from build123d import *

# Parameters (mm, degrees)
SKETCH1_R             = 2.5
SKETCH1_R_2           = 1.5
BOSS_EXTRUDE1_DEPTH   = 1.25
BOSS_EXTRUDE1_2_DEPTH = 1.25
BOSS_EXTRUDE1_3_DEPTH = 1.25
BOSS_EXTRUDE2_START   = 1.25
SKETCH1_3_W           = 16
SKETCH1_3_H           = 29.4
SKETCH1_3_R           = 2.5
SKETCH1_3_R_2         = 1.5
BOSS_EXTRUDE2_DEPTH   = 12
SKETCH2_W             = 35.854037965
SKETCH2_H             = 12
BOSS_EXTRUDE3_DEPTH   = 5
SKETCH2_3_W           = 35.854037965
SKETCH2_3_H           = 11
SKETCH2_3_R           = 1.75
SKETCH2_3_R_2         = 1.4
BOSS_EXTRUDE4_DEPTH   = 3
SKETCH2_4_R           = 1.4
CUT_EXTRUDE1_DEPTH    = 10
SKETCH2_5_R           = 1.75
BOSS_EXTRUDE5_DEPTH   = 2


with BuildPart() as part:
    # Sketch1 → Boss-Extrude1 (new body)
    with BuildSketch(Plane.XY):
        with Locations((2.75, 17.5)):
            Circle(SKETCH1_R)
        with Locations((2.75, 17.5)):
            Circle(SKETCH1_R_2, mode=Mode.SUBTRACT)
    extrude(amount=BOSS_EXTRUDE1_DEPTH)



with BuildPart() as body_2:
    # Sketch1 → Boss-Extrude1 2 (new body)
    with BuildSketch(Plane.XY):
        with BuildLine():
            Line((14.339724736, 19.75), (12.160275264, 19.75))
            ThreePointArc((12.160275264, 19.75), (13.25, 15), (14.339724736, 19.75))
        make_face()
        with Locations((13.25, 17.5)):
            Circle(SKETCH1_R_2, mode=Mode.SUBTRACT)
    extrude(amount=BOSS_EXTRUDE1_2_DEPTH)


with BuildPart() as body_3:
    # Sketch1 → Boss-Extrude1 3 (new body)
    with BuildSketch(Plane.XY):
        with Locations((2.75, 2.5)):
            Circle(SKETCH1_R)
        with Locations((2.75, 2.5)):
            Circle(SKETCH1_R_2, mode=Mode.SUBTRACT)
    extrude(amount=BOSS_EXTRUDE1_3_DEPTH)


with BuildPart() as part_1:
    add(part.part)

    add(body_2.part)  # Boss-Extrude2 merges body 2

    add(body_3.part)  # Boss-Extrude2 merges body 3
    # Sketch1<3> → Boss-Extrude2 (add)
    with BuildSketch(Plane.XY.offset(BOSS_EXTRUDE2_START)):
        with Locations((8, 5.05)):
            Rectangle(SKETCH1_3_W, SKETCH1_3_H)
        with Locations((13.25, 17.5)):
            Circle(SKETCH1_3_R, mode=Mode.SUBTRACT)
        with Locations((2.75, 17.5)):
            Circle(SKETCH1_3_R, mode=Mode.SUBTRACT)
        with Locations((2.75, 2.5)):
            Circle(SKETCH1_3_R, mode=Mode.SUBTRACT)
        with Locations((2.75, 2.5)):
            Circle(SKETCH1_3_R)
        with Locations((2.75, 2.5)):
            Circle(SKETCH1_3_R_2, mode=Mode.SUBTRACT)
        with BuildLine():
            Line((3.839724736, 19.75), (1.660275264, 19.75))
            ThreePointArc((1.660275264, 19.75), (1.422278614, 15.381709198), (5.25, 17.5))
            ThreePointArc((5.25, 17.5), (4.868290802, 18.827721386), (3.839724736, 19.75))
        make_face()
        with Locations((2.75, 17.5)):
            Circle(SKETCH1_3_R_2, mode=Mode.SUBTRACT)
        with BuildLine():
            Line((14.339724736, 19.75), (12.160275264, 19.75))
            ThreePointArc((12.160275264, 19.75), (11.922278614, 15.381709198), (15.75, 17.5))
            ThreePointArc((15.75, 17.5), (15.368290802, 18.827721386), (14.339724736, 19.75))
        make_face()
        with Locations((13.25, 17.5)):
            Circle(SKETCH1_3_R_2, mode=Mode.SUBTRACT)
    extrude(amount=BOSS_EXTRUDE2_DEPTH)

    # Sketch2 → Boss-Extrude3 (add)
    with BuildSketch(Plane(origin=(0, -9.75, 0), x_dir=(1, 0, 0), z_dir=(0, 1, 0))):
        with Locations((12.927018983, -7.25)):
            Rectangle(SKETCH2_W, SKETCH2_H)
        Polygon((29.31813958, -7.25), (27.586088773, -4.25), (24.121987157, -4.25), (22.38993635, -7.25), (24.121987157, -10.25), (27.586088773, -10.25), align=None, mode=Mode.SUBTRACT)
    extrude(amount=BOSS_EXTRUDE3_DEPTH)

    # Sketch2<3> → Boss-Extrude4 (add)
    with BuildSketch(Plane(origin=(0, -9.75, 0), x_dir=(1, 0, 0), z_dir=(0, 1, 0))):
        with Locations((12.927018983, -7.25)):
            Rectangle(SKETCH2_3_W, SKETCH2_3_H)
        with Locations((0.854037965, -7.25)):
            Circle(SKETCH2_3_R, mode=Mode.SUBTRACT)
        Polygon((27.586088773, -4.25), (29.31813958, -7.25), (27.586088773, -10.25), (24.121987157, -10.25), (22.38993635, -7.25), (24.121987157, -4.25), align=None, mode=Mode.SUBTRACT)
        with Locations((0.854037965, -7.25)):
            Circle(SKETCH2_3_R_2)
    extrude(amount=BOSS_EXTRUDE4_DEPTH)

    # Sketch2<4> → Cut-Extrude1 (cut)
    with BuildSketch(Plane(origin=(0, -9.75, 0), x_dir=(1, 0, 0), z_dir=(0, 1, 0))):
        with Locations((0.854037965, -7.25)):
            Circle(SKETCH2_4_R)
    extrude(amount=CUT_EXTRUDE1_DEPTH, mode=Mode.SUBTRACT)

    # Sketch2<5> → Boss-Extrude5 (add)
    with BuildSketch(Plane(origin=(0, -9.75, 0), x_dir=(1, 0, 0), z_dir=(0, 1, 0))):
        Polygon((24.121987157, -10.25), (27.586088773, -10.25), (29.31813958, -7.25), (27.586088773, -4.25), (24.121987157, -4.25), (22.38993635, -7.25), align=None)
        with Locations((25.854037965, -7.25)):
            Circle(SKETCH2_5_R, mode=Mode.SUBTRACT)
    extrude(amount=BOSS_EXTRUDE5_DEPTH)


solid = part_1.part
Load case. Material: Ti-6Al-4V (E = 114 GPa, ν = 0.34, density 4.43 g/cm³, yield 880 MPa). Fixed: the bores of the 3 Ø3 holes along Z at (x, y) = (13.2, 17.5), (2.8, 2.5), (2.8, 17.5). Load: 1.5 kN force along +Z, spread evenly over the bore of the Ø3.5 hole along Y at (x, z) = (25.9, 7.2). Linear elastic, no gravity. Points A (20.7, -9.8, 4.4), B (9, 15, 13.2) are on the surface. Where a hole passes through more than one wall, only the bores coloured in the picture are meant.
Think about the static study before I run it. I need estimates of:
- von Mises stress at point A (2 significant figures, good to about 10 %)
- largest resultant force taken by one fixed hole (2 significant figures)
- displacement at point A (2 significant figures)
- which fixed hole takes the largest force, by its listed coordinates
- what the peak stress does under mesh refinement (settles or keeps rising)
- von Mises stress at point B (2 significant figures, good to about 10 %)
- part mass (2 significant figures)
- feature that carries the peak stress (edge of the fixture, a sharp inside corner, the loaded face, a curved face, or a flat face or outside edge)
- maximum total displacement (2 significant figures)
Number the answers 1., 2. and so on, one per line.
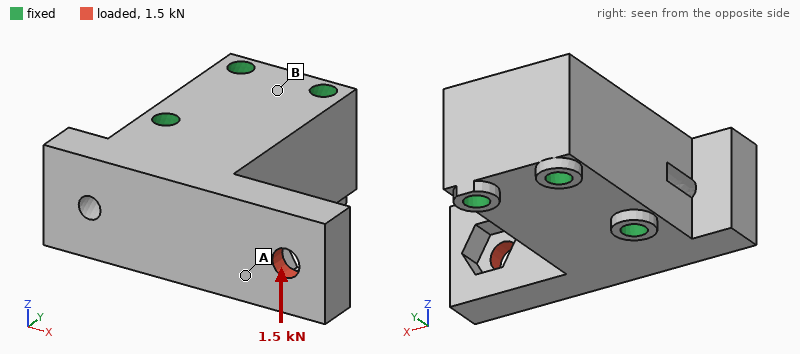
1. 83 MPa
2. 1.2 kN
3. 46 µm
4. (2.8, 2.5)
5. keeps rising
6. 22 MPa
7. 29 g
8. edge of the fixture
9. 93 µm
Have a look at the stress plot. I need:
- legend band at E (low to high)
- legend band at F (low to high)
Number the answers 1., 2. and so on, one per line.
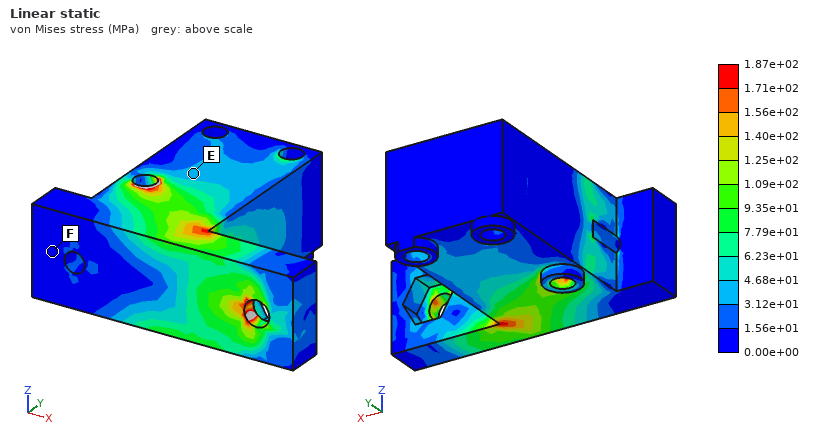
1. 3.12e+01 to 4.68e+01 MPa
2. 0.00e+00 to 1.56e+01 MPa
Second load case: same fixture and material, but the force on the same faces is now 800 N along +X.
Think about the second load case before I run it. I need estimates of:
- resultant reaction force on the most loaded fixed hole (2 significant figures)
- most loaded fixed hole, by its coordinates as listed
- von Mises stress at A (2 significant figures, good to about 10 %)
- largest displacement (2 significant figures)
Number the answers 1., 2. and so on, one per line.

1. 1.1 kN
2. (2.8, 2.5)
3. 39 MPa
4. 21 µm
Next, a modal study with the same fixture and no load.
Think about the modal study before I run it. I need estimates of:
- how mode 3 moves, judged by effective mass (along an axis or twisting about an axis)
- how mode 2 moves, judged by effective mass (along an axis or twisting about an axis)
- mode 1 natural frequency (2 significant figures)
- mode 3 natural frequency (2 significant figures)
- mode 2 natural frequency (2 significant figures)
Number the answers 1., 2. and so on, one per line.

1. along X
2. along Z
3. 12 kHz
4. 27 kHz
5. 14 kHz
